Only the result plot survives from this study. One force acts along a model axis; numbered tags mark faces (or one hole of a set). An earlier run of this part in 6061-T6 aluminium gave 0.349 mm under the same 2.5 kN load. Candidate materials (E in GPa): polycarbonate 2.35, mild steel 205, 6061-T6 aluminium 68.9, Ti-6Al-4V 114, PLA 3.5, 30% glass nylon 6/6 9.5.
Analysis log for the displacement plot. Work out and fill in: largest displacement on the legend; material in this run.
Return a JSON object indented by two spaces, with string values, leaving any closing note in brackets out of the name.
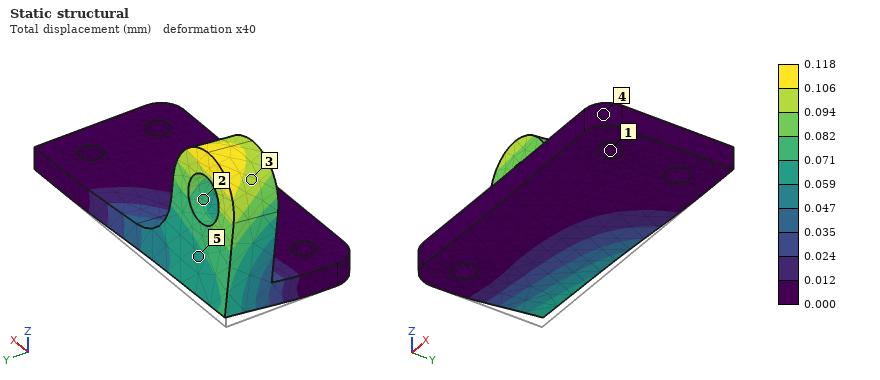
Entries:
{
  "largest displacement on the legend": "0.118 mm",
  "material in this run": "mild steel"
}
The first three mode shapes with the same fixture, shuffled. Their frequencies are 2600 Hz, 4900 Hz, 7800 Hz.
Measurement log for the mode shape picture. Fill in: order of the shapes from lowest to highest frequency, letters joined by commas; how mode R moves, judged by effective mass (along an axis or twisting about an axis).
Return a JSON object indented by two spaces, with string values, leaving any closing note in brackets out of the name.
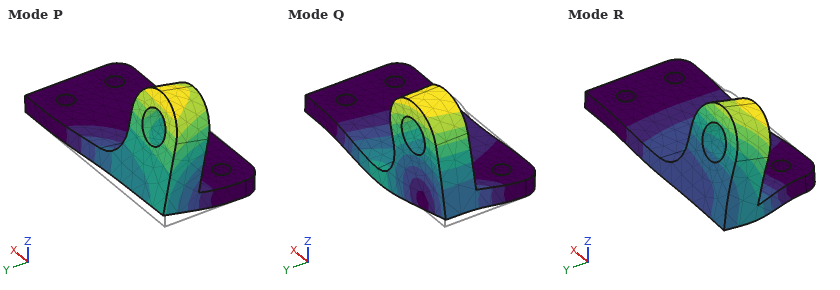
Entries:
{
  "order of the shapes from lowest to highest frequency, letters joined by commas": "P, Q, R",
  "how mode R moves, judged by effective mass": "along Z"
}
